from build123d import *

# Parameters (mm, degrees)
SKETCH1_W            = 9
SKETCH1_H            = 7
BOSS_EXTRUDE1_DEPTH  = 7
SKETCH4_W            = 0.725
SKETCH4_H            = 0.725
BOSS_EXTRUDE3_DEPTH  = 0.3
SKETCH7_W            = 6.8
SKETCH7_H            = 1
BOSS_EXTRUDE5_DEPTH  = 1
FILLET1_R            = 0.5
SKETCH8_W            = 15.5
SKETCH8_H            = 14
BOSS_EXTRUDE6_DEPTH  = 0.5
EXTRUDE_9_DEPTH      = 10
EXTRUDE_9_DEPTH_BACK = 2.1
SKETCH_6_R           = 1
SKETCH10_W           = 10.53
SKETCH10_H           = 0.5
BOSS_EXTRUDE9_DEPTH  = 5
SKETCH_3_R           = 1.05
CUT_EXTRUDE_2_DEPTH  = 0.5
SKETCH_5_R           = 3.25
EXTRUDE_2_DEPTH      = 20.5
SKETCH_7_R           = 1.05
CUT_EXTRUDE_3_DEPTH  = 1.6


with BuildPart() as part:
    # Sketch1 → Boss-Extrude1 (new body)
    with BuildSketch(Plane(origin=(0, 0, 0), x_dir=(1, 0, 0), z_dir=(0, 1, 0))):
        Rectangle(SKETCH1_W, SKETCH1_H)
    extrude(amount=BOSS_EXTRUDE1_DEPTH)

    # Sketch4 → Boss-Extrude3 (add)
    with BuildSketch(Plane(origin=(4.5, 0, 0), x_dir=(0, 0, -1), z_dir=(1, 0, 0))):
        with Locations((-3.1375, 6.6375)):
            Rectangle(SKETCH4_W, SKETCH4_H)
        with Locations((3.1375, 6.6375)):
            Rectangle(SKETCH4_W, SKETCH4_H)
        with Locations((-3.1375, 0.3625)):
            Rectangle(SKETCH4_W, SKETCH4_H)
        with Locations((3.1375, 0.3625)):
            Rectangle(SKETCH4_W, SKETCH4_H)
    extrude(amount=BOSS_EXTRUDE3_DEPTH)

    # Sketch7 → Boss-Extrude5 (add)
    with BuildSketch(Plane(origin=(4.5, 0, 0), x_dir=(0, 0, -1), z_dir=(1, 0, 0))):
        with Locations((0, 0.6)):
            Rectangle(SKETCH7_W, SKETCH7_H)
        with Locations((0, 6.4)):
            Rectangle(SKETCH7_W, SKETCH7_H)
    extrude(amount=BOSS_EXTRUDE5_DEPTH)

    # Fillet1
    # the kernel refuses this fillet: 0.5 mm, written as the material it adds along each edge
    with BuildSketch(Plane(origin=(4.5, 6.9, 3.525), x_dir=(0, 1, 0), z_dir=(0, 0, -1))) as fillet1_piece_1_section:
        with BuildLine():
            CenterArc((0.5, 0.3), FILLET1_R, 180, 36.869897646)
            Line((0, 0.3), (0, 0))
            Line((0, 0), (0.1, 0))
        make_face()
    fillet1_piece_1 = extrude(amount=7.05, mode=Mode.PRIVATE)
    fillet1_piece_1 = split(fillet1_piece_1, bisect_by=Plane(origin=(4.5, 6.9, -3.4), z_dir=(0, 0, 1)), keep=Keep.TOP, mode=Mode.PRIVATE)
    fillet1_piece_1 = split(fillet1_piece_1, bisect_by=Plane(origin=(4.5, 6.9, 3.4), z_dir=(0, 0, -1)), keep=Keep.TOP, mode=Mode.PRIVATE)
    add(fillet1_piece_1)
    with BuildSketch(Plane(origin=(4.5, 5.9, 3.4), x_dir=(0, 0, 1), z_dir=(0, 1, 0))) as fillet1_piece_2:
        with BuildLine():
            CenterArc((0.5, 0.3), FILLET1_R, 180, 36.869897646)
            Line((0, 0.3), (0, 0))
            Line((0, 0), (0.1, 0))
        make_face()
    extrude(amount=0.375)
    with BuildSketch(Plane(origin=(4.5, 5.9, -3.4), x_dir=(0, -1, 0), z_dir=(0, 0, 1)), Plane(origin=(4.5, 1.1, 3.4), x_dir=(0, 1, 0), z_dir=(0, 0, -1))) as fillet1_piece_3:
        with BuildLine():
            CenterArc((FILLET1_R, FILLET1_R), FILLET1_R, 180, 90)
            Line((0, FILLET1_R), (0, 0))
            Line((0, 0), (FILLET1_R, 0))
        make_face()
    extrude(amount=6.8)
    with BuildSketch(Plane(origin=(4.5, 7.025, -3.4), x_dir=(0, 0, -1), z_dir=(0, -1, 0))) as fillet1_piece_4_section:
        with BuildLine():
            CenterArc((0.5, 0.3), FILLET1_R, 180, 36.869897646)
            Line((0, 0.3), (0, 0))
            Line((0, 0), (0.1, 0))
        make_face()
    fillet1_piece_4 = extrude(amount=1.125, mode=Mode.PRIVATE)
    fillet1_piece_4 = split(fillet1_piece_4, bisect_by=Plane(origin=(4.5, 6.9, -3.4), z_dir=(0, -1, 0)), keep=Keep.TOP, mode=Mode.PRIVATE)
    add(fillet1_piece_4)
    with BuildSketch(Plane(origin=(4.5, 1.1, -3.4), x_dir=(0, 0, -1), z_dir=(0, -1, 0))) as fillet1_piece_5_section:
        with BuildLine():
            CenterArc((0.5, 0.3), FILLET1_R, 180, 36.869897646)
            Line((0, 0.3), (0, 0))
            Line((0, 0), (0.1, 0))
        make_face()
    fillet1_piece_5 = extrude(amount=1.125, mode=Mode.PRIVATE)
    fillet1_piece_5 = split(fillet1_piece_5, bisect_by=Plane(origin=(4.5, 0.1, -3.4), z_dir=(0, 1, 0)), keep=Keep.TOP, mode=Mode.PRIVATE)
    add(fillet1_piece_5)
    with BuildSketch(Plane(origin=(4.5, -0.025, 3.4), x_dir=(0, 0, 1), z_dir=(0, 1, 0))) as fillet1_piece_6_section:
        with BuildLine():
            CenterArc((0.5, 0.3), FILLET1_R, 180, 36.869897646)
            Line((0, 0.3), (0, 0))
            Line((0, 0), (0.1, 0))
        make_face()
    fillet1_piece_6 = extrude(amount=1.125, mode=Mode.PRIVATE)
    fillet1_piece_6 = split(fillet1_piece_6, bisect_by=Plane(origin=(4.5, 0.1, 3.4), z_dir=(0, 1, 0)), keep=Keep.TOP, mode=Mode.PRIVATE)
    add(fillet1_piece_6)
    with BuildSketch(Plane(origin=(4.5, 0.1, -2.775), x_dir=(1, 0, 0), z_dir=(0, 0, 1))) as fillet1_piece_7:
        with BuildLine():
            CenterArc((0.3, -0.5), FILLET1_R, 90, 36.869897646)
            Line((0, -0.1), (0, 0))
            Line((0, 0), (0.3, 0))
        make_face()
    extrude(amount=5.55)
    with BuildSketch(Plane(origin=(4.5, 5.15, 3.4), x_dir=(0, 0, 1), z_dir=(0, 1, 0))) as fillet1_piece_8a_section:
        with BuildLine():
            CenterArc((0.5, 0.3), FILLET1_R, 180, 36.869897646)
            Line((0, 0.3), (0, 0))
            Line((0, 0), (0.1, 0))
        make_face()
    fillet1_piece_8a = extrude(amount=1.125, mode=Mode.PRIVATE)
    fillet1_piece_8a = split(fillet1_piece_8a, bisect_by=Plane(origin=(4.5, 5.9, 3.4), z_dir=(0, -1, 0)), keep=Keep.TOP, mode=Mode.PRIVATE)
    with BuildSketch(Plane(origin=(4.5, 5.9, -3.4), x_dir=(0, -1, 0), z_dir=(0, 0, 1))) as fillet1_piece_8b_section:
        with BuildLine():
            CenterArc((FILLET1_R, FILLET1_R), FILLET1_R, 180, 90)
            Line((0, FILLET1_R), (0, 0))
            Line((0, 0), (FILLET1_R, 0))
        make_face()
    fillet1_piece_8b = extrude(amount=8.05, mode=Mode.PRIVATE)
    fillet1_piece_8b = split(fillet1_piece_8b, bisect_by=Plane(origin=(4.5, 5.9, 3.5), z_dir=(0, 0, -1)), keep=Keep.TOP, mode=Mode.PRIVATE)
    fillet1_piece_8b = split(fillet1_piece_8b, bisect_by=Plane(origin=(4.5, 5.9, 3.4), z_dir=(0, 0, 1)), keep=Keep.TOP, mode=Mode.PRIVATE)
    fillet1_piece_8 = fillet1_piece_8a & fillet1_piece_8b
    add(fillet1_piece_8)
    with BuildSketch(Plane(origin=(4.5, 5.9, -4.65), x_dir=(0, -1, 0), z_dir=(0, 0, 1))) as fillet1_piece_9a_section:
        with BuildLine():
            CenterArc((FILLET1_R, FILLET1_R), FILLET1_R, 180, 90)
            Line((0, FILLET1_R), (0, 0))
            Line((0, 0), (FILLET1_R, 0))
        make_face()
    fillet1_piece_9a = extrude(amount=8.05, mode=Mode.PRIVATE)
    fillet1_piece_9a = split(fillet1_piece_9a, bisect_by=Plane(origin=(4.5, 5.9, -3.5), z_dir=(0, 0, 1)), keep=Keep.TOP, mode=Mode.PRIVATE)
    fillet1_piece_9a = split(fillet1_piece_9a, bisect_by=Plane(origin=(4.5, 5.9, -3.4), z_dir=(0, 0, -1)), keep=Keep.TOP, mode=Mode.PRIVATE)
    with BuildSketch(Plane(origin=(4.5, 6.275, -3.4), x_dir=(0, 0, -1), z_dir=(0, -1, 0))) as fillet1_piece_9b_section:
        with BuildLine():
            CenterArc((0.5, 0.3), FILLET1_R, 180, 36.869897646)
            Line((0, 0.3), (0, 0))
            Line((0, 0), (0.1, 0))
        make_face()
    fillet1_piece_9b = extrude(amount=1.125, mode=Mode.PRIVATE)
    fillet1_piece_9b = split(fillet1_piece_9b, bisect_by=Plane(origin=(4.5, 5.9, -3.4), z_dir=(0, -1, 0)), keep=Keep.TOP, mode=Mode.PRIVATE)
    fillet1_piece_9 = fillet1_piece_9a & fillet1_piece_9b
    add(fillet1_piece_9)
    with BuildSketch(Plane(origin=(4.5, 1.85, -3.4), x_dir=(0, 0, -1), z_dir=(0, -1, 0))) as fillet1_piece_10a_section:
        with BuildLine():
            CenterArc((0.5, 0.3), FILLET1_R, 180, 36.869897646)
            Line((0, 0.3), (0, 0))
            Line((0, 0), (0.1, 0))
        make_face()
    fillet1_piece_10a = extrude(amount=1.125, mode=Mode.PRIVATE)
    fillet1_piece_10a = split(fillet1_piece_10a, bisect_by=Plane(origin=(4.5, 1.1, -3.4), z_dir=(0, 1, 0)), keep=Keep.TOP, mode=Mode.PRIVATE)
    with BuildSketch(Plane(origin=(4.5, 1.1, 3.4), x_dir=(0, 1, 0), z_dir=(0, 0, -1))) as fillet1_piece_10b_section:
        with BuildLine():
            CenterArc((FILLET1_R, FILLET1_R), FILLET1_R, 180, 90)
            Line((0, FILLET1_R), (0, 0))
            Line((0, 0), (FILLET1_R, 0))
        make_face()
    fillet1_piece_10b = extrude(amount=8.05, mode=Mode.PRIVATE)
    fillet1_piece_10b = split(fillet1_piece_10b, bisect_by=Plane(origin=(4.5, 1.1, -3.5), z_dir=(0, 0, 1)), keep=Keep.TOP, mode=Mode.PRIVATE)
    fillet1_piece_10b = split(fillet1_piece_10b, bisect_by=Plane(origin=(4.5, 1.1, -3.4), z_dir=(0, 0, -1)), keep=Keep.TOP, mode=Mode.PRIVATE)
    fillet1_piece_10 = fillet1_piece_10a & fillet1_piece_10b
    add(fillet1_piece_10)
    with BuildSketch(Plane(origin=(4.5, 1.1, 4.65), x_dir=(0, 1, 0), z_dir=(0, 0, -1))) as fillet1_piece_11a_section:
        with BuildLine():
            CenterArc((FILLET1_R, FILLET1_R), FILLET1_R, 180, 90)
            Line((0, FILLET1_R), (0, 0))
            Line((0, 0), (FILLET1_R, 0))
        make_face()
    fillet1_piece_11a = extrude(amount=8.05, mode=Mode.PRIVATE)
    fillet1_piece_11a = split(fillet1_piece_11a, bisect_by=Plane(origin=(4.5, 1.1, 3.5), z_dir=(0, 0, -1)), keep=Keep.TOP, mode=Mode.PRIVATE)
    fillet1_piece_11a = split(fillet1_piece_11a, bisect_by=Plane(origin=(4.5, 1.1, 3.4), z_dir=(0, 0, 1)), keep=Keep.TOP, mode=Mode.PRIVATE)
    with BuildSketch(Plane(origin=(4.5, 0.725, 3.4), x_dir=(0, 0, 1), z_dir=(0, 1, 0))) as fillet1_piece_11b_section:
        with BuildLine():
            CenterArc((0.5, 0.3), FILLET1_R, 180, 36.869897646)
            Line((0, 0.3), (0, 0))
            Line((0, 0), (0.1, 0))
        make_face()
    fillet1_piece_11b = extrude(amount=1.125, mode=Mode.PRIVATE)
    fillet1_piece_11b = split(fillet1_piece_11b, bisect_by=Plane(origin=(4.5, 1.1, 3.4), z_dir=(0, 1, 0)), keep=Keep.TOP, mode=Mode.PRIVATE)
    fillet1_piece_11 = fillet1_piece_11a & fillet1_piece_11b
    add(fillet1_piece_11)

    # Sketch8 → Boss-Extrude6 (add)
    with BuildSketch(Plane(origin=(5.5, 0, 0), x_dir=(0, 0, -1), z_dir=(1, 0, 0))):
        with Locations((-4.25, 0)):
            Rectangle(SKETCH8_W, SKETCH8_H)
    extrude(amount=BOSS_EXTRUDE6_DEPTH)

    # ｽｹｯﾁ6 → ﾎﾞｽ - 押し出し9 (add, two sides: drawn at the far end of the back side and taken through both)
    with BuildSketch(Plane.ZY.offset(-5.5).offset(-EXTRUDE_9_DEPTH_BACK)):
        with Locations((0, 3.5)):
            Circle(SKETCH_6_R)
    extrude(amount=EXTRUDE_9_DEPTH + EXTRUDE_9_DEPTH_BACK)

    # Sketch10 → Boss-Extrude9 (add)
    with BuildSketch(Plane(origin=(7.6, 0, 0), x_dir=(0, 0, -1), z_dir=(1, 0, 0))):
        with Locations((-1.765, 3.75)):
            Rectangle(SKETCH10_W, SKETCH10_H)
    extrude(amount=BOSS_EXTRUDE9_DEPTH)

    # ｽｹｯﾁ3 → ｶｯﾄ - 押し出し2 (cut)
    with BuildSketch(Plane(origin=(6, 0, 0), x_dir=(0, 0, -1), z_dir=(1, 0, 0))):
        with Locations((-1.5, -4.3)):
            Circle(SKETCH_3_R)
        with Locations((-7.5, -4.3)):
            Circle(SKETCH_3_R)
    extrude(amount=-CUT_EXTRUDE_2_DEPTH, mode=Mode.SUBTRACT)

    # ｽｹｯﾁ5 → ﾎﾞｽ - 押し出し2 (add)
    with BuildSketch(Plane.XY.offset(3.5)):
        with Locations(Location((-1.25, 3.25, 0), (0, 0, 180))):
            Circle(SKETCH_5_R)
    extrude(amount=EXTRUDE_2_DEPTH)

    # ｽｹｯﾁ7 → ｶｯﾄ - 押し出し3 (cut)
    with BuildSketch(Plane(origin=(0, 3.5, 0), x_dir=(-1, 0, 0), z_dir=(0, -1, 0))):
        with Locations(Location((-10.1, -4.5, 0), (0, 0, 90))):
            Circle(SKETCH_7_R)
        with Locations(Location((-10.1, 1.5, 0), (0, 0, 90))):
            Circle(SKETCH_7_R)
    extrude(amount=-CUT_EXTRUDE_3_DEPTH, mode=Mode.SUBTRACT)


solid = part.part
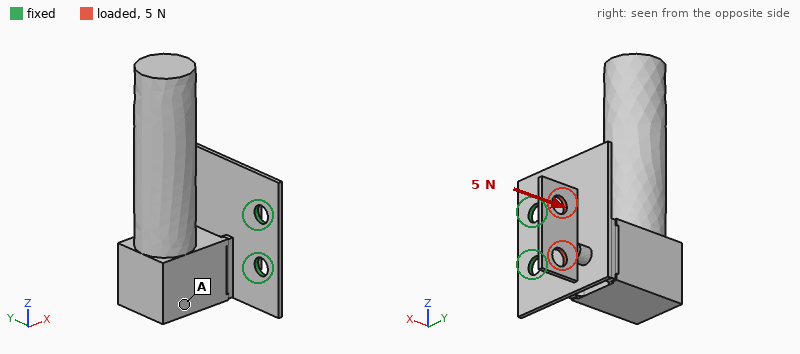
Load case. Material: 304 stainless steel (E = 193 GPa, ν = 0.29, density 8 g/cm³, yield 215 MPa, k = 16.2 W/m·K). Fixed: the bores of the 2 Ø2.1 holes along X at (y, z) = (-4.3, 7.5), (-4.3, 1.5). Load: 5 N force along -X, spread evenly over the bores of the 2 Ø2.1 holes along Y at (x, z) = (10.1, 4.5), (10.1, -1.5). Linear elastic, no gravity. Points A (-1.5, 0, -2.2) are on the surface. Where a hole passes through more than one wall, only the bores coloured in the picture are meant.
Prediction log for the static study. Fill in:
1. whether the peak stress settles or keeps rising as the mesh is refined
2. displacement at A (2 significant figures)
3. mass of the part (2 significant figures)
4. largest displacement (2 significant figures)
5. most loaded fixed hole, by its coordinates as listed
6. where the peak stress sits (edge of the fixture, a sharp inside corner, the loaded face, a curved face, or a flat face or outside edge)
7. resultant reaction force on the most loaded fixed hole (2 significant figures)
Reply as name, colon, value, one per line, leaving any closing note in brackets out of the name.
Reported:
whether the peak stress settles or keeps rising as the mesh is refined: keeps rising
displacement at A: 32 µm
mass of the part: 10 g
largest displacement: 60 µm
most loaded fixed hole, by its coordinates as listed: (-4.3, 1.5)
where the peak stress sits: edge of the fixture
resultant reaction force on the most loaded fixed hole: 4.1 N
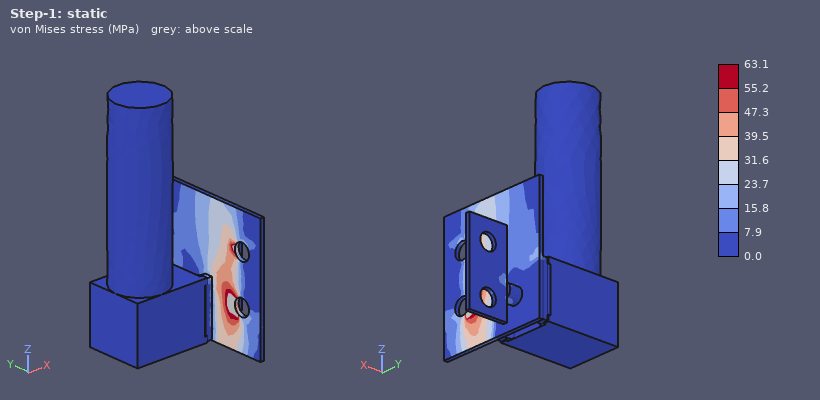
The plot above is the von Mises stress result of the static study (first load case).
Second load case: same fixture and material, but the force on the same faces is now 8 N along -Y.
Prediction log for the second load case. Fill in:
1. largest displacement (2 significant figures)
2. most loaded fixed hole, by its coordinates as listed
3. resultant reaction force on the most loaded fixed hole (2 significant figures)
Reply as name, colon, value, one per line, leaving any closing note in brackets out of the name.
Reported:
largest displacement: 99 µm
most loaded fixed hole, by its coordinates as listed: (-4.3, 1.5)
resultant reaction force on the most loaded fixed hole: 7.0 N
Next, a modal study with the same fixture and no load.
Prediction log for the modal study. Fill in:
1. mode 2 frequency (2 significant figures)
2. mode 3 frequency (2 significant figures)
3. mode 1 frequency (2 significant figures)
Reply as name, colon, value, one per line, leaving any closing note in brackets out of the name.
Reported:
mode 2 frequency: 600 Hz
mode 3 frequency: 3400 Hz
mode 1 frequency: 490 Hz
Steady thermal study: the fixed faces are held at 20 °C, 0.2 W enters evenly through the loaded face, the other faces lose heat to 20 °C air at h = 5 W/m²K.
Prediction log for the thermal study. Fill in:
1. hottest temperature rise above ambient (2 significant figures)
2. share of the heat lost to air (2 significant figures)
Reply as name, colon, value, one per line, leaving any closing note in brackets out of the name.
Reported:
hottest temperature rise above ambient: 42 K
share of the heat lost to air: 30 %
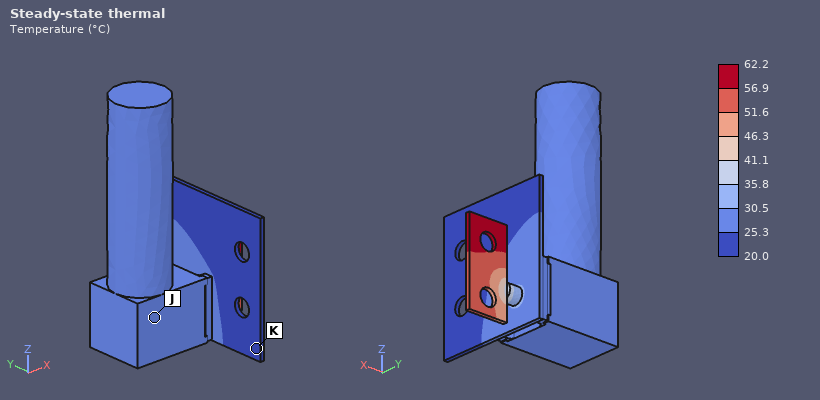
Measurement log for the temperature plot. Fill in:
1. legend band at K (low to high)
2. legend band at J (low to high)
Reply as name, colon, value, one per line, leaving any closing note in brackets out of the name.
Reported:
legend band at K: 20.0 to 25.3 °C
legend band at J: 25.3 to 30.5 °C
